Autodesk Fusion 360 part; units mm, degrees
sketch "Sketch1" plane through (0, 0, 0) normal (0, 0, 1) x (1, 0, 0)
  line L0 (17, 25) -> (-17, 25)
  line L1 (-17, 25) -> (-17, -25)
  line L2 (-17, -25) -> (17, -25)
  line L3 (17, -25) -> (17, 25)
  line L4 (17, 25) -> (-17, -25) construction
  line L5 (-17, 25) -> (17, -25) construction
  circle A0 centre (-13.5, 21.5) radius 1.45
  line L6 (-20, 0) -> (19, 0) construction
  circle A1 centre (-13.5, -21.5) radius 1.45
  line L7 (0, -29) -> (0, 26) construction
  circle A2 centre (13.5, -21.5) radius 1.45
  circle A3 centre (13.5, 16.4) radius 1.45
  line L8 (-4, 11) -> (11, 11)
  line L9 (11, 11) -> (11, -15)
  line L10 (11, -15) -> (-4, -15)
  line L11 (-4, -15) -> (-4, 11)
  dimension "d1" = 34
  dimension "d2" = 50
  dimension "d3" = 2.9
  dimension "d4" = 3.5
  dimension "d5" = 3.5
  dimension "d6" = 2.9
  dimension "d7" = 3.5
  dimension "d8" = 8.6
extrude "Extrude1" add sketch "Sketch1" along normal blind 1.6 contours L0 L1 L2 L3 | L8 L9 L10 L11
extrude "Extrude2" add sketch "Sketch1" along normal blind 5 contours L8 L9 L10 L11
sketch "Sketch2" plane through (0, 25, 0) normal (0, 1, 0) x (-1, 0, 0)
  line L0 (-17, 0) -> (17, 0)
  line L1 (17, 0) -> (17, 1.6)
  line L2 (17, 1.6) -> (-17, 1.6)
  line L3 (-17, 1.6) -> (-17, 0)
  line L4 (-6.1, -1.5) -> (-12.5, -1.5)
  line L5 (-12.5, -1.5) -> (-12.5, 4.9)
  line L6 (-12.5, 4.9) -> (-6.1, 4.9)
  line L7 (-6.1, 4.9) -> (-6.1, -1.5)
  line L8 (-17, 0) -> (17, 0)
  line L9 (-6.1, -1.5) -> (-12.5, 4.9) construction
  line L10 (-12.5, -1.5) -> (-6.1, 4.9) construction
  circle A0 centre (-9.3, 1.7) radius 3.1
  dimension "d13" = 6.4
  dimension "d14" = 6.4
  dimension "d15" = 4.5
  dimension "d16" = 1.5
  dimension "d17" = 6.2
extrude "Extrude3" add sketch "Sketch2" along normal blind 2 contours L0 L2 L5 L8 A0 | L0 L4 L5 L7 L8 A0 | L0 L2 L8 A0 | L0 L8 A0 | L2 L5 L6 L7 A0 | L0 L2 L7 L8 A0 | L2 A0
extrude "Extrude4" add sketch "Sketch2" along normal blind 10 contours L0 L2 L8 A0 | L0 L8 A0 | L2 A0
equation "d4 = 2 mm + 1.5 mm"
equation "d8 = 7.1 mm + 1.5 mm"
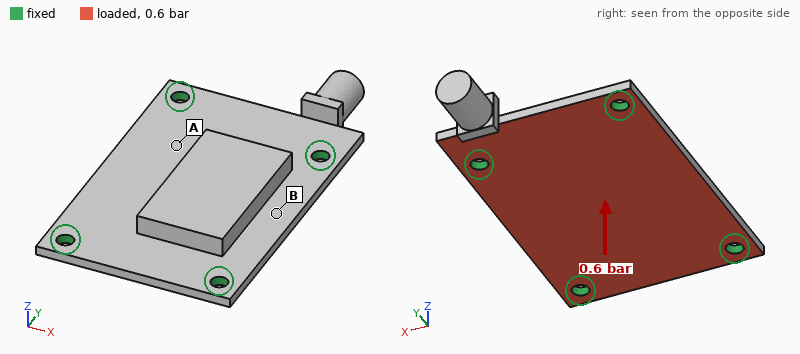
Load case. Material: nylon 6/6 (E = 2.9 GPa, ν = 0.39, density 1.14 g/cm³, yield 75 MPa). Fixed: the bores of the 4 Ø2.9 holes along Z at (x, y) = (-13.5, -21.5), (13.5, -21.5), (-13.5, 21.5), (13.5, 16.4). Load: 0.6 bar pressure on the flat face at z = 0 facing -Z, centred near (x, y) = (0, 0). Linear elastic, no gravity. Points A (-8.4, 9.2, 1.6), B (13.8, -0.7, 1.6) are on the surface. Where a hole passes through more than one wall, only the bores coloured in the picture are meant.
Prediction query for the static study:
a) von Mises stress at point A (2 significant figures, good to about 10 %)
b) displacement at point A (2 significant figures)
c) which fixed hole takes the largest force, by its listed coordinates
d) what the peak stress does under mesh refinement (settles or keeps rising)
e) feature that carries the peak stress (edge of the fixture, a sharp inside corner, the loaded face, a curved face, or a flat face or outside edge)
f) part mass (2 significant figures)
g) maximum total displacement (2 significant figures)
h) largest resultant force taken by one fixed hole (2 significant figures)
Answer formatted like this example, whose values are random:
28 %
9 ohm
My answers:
6.7 MPa
0.23 mm
(13.5, 16.4)
keeps rising
edge of the fixture
4.9 g
0.39 mm
35 N
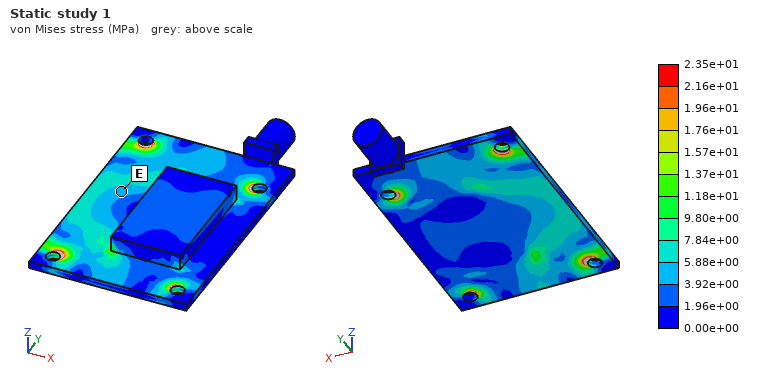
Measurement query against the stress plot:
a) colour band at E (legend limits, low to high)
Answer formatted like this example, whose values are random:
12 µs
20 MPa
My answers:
3.92e+00 to 5.88e+00 MPa
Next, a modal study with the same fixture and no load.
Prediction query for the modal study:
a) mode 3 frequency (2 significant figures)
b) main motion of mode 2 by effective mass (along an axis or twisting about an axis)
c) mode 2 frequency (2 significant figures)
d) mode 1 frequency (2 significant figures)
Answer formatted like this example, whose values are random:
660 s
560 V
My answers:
2800 Hz
along Z
1700 Hz
1100 Hz
